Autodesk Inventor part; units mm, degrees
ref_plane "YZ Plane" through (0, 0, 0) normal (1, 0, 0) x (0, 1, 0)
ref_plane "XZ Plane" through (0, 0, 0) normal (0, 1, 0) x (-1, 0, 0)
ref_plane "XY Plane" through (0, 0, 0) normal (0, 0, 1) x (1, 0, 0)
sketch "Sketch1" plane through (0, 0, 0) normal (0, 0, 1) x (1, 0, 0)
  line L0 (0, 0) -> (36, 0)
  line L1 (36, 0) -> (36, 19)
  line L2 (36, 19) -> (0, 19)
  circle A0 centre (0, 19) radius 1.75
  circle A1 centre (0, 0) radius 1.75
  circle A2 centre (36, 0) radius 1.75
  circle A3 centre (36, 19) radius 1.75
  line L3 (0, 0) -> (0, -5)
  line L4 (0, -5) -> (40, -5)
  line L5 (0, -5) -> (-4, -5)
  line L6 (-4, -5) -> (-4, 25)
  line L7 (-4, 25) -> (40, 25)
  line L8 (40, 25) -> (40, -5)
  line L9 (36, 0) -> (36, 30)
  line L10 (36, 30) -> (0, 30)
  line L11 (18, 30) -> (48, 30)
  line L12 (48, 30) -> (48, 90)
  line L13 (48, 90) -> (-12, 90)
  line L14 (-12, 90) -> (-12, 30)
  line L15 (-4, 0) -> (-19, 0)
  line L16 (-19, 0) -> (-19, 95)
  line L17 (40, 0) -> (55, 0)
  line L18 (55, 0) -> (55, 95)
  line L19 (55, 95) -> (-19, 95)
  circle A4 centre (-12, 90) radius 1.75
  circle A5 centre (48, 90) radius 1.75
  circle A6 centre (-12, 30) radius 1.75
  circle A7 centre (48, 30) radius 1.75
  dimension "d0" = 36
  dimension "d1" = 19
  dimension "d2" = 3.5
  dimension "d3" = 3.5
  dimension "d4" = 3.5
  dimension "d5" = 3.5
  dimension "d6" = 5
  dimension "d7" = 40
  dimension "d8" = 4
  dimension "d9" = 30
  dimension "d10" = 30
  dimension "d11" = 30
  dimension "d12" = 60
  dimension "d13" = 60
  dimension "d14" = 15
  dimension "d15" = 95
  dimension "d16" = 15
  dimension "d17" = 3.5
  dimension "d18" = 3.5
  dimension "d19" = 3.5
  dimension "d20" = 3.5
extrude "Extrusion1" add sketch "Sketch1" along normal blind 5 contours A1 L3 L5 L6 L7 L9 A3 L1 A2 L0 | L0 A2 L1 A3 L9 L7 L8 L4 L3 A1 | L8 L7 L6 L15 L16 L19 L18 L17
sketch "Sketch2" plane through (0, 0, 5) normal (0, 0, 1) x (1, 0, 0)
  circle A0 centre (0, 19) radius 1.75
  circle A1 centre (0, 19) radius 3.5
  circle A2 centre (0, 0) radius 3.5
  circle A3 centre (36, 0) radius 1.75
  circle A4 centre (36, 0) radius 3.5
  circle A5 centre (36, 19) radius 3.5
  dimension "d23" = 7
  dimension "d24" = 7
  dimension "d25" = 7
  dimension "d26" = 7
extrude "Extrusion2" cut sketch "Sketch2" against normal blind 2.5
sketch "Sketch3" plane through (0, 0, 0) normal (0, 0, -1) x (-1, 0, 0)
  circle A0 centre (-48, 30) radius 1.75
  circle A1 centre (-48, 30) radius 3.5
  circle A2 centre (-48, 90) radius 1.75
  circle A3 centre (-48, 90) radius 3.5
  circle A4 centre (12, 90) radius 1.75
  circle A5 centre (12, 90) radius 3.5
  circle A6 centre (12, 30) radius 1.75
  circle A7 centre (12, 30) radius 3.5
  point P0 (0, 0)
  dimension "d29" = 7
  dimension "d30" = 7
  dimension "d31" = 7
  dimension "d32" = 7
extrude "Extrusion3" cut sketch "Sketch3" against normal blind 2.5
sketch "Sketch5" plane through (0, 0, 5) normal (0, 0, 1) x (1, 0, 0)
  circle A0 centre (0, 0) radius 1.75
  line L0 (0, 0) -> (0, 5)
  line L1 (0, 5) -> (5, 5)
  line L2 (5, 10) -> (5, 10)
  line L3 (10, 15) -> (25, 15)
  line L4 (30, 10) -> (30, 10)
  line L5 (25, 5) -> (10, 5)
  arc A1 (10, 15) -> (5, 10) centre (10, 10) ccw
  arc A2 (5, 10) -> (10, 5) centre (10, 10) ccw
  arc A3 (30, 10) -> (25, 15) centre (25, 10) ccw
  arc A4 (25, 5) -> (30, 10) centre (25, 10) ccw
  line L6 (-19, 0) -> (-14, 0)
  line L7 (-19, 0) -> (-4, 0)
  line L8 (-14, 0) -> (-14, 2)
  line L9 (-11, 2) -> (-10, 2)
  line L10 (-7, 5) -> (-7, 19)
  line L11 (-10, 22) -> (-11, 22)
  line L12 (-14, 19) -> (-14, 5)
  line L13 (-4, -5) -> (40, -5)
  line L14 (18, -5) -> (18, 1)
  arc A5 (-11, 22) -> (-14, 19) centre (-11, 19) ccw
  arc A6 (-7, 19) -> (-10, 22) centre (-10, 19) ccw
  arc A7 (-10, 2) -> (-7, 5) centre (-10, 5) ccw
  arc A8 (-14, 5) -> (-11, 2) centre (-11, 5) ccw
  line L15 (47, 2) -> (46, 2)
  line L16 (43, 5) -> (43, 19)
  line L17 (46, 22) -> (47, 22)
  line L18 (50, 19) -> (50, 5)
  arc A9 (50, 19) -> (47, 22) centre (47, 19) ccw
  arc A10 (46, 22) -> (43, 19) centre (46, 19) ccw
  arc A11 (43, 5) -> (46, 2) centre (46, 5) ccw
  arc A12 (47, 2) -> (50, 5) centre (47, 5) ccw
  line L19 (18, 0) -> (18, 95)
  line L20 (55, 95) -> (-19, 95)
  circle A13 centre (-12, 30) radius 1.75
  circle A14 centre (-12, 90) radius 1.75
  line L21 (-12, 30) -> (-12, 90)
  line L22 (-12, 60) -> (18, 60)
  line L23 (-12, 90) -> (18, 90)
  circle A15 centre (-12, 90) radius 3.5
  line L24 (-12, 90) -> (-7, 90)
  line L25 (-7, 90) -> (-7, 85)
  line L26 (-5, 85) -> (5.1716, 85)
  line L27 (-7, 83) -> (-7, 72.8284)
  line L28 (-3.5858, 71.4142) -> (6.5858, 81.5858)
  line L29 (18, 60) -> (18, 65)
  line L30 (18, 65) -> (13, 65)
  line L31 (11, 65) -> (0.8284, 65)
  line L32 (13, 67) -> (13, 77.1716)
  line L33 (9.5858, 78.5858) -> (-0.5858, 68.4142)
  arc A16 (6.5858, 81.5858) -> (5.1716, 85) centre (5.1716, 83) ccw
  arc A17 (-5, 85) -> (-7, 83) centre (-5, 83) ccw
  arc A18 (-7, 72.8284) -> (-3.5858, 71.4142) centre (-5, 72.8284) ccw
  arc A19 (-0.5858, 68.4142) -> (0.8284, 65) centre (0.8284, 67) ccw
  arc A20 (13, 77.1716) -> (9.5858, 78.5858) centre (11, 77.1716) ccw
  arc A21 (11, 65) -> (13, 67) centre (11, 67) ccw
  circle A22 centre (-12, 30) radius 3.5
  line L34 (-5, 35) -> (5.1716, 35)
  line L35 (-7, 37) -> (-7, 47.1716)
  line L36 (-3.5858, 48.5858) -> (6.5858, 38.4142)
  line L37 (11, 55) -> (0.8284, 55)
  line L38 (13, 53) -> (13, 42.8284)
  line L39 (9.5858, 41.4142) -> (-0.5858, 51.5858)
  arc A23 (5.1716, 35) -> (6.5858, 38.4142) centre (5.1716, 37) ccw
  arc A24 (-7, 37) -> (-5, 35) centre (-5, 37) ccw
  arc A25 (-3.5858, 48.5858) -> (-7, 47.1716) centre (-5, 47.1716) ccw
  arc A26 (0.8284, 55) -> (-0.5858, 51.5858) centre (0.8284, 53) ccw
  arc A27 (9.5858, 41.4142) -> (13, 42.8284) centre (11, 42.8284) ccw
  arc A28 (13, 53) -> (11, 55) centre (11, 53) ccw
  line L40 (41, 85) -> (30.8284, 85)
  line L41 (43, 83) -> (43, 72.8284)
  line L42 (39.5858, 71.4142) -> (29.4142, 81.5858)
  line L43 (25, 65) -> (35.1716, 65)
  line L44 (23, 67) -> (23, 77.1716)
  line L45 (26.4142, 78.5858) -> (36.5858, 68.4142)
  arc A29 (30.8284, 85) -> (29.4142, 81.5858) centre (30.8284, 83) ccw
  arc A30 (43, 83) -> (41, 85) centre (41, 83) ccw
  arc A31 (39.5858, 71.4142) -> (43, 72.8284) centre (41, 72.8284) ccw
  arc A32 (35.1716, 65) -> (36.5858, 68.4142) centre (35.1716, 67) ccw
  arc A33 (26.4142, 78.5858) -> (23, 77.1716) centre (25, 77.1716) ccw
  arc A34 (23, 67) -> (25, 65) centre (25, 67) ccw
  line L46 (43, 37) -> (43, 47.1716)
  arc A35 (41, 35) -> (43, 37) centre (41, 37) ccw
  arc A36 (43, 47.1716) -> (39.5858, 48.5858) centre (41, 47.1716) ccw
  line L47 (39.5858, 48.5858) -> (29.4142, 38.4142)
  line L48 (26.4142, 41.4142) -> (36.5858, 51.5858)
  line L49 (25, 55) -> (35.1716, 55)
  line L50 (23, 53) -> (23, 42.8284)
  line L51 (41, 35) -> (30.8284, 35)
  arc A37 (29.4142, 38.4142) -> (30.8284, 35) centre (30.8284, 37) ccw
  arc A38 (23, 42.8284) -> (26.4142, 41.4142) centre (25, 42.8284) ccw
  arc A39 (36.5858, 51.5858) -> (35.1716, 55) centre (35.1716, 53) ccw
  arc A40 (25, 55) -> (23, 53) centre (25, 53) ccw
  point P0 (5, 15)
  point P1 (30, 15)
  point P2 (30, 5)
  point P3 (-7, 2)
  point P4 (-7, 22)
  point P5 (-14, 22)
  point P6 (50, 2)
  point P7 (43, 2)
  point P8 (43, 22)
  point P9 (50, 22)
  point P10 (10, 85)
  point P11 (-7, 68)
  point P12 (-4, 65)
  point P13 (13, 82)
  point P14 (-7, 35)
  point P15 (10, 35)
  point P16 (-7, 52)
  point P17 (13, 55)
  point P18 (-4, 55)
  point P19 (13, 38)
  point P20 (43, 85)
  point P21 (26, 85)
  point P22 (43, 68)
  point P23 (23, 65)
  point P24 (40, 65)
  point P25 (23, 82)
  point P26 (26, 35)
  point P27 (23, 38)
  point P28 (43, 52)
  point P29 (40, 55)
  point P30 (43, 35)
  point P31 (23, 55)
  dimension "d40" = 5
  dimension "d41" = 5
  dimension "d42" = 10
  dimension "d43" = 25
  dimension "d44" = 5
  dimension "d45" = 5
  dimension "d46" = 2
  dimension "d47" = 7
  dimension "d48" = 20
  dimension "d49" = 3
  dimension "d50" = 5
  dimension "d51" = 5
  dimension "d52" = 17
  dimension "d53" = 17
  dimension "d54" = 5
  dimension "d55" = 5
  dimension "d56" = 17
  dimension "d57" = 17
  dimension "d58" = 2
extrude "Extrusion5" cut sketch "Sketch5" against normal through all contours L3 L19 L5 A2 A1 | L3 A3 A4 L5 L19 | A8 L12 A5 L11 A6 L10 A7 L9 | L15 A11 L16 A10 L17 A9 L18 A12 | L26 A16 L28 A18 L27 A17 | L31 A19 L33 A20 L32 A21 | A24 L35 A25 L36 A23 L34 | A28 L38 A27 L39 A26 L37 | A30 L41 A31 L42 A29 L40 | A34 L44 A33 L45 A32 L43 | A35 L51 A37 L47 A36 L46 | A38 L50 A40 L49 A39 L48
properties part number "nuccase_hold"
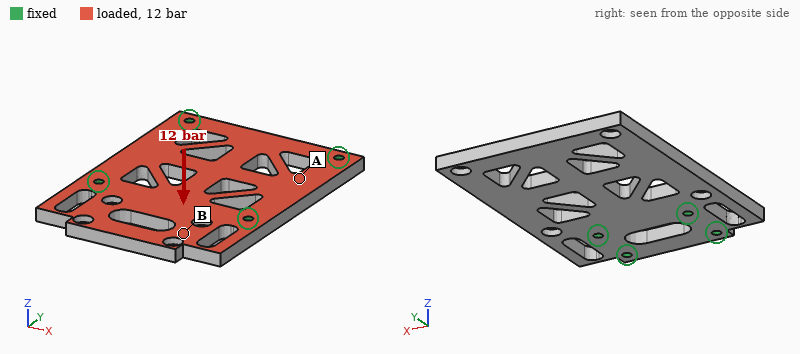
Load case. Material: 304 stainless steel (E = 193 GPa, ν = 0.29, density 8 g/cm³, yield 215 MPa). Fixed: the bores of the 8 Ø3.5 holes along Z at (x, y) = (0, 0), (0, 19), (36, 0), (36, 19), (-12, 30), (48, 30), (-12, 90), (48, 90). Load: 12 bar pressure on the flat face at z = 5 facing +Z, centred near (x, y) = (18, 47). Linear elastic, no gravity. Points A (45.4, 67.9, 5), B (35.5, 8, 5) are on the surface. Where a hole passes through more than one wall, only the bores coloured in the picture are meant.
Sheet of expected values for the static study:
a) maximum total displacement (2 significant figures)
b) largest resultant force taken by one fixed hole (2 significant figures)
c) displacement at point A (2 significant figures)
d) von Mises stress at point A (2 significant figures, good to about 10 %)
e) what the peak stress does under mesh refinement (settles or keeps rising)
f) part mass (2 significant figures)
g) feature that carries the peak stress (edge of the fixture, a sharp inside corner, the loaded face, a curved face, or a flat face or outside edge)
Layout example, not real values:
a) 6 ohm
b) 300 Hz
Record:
a) 78 µm
b) 1.5 kN
c) 46 µm
d) 69 MPa
e) keeps rising
f) 220 g
g) edge of the fixture
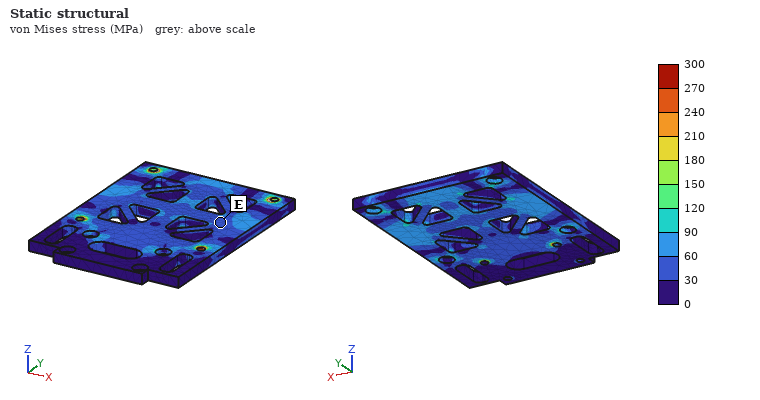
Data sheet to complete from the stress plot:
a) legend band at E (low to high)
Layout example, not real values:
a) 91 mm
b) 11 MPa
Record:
a) 30 to 60 MPa
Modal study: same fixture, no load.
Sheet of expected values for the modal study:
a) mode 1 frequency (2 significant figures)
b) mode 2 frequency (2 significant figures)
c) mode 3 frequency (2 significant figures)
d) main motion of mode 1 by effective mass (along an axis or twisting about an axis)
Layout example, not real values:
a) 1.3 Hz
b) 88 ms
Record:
a) 3800 Hz
b) 5700 Hz
c) 5900 Hz
d) along Z
